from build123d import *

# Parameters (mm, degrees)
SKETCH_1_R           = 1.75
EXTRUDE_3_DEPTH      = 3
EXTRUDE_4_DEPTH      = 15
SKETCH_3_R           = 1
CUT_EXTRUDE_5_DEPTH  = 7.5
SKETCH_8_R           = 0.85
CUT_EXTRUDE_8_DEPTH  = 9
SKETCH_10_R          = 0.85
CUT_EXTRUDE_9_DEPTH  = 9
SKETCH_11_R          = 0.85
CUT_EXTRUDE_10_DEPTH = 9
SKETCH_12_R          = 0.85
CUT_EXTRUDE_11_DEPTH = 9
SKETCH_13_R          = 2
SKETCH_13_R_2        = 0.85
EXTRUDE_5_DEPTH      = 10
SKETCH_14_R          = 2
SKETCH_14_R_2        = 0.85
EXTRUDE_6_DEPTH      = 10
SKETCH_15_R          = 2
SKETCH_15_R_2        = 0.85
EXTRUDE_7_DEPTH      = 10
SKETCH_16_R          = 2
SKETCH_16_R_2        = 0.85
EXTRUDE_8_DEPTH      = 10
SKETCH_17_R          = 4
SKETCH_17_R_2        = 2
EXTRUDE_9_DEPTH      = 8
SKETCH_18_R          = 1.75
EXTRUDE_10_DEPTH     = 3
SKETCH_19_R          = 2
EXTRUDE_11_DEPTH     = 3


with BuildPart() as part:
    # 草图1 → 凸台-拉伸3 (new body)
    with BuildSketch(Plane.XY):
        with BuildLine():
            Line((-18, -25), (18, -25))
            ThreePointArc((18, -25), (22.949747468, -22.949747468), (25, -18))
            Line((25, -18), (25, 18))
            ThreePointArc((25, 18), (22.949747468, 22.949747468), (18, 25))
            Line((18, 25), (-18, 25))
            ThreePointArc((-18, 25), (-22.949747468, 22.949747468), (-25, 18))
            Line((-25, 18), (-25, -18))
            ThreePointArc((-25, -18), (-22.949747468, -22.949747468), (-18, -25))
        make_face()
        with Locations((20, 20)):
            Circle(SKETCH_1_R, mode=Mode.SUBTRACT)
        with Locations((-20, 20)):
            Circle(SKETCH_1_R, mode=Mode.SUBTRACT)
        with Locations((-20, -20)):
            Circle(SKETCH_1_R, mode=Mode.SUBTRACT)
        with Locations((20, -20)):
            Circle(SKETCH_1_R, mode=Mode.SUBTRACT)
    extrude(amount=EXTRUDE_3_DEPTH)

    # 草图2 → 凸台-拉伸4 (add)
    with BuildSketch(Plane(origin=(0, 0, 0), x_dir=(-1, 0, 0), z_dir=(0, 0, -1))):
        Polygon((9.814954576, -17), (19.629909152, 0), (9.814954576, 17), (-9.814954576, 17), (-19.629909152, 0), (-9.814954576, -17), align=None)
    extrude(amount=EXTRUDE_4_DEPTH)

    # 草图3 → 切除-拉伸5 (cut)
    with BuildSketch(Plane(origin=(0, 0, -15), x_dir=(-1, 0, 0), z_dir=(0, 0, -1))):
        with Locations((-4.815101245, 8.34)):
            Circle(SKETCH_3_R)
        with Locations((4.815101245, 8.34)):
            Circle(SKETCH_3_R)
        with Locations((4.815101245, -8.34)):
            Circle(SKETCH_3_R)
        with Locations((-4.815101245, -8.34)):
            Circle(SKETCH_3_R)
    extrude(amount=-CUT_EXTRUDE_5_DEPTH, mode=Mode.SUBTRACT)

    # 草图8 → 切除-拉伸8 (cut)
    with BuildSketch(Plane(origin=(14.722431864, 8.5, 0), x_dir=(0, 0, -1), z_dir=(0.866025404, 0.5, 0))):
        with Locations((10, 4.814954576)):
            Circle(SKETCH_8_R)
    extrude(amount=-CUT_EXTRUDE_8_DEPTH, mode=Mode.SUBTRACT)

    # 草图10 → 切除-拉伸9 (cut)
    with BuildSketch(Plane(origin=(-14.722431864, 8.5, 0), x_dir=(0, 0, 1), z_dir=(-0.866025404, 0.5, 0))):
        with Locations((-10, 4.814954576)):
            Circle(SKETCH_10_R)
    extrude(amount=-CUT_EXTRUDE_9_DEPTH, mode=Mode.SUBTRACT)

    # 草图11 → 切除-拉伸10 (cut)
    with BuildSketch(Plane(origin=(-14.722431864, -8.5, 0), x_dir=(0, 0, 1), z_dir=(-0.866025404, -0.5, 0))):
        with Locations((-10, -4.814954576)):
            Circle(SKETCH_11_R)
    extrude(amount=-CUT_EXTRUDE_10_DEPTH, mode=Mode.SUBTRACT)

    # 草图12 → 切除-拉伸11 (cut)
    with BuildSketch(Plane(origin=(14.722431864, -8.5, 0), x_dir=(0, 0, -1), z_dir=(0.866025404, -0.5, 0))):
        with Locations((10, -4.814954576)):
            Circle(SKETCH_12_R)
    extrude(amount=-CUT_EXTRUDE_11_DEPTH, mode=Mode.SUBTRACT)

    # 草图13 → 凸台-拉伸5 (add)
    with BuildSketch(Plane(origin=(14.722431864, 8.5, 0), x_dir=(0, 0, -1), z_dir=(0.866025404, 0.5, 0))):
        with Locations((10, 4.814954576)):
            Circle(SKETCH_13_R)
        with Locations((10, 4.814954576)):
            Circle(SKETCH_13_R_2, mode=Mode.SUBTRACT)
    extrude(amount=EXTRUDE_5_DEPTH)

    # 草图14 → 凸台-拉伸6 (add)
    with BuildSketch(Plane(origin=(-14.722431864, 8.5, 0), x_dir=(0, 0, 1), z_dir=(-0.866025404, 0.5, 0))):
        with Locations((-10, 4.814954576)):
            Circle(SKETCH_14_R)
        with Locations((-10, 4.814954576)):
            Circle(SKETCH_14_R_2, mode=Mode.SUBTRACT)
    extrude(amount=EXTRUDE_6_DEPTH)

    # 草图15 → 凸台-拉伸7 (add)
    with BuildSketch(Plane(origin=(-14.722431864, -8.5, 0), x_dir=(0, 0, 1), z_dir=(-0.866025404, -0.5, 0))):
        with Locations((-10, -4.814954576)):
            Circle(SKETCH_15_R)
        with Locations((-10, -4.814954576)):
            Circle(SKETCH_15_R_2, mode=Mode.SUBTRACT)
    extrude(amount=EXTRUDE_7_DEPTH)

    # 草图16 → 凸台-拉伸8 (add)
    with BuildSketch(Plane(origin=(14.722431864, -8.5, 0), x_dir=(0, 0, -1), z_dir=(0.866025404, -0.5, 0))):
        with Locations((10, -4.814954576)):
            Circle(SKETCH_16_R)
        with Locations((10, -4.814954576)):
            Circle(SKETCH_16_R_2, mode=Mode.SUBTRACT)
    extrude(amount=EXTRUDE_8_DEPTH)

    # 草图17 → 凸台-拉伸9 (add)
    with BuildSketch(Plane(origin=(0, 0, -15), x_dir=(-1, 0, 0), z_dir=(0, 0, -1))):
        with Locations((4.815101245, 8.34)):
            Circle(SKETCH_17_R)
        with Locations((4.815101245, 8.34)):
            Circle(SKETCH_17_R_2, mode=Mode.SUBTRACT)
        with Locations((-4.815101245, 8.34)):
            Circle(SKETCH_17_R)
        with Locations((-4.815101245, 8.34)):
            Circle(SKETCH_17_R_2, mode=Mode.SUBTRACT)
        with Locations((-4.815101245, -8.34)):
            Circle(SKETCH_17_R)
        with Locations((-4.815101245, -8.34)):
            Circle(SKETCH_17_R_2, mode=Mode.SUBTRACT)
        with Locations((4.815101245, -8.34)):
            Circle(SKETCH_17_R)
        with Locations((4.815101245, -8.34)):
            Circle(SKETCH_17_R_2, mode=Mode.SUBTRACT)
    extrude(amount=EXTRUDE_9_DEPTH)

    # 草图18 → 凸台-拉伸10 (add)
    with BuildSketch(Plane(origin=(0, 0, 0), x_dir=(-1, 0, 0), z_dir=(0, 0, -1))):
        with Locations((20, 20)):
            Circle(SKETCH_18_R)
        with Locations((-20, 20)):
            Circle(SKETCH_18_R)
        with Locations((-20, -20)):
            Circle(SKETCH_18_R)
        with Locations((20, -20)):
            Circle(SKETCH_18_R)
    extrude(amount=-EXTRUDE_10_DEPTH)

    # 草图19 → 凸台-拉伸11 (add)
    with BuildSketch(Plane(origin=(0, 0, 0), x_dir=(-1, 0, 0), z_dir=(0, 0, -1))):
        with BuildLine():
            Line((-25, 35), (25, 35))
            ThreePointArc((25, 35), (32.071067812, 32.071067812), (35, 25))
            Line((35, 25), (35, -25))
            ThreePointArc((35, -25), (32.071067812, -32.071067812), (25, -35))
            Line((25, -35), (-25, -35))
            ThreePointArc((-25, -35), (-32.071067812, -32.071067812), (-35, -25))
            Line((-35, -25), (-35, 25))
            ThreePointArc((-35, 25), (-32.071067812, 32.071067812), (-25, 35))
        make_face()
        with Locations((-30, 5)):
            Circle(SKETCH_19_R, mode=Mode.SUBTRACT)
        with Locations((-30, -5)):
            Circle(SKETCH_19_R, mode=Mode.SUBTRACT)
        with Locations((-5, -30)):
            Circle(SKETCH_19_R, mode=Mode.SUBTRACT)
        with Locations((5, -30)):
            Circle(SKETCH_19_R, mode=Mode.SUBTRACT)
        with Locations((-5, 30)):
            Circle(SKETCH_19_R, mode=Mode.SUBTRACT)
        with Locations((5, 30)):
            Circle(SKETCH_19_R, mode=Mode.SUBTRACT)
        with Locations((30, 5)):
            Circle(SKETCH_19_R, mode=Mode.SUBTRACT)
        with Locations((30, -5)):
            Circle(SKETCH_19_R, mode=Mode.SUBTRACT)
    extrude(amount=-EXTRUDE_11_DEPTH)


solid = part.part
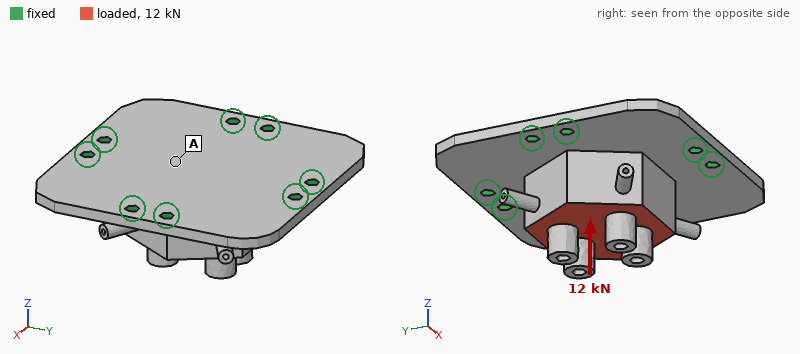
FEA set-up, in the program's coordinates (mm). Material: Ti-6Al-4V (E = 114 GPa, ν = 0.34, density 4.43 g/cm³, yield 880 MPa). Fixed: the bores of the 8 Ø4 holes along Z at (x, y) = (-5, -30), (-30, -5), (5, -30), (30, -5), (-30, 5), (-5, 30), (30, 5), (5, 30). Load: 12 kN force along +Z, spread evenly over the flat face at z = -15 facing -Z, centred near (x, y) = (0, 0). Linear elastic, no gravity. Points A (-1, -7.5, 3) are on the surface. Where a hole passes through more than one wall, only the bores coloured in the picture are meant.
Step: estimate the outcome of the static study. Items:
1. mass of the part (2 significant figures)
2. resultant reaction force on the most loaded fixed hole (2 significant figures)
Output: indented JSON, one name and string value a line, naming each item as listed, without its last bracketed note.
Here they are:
{
  "mass of the part": "140 g",
  "resultant reaction force on the most loaded fixed hole": "1.7 kN"
}
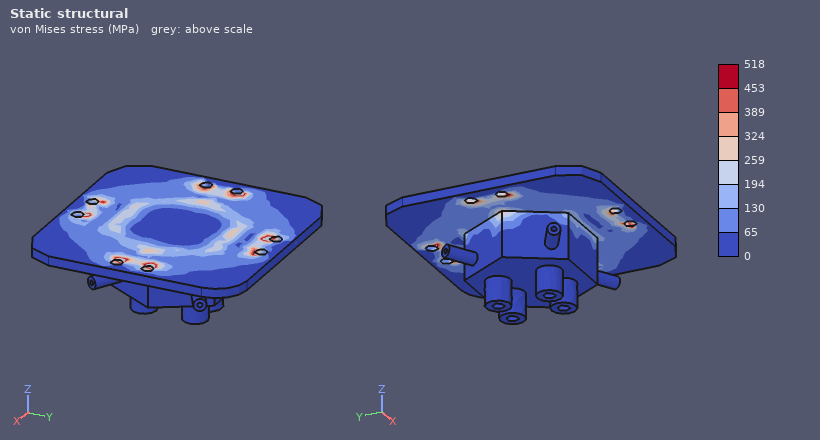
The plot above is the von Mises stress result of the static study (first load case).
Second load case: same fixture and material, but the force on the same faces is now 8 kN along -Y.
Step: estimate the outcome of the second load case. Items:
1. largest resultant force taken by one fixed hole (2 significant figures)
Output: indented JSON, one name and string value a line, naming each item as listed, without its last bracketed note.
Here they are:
{
  "largest resultant force taken by one fixed hole": "2.0 kN"
}
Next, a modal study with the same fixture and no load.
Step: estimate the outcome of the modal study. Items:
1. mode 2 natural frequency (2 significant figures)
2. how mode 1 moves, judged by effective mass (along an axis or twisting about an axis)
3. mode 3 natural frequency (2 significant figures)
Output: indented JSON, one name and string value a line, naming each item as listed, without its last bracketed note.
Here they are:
{
  "mode 2 natural frequency": "6500 Hz",
  "how mode 1 moves, judged by effective mass": "along Z",
  "mode 3 natural frequency": "6600 Hz"
}
